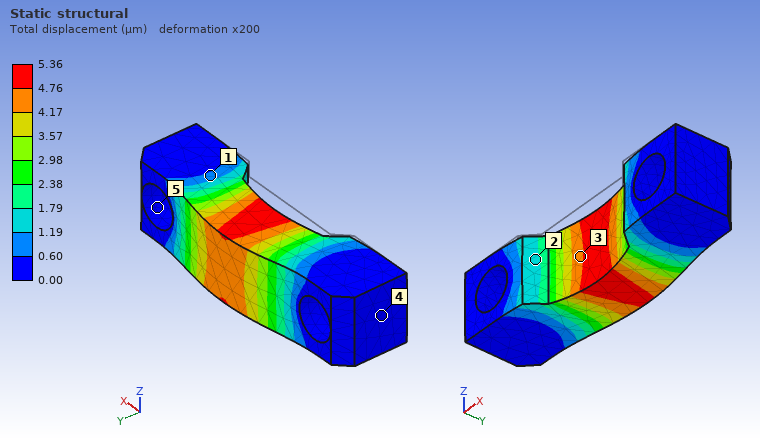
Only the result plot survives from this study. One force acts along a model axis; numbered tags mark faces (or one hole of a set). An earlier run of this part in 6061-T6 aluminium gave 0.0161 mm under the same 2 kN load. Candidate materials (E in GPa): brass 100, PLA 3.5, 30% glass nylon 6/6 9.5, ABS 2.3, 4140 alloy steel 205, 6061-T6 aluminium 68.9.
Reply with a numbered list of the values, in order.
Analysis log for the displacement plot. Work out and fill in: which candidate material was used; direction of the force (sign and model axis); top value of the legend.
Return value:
1. 4140 alloy steel
2. +Y
3. 5.36 µm
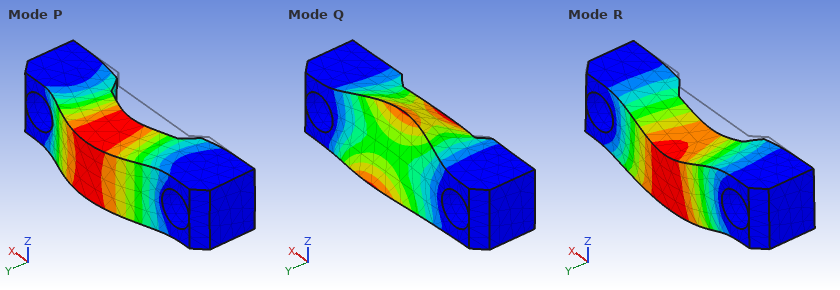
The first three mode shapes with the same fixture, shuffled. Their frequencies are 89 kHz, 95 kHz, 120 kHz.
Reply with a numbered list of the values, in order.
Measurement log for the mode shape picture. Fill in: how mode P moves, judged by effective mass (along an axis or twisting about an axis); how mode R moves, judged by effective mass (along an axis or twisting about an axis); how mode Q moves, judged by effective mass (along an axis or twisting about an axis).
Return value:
1. along Y
2. along Z
3. twisting about X
